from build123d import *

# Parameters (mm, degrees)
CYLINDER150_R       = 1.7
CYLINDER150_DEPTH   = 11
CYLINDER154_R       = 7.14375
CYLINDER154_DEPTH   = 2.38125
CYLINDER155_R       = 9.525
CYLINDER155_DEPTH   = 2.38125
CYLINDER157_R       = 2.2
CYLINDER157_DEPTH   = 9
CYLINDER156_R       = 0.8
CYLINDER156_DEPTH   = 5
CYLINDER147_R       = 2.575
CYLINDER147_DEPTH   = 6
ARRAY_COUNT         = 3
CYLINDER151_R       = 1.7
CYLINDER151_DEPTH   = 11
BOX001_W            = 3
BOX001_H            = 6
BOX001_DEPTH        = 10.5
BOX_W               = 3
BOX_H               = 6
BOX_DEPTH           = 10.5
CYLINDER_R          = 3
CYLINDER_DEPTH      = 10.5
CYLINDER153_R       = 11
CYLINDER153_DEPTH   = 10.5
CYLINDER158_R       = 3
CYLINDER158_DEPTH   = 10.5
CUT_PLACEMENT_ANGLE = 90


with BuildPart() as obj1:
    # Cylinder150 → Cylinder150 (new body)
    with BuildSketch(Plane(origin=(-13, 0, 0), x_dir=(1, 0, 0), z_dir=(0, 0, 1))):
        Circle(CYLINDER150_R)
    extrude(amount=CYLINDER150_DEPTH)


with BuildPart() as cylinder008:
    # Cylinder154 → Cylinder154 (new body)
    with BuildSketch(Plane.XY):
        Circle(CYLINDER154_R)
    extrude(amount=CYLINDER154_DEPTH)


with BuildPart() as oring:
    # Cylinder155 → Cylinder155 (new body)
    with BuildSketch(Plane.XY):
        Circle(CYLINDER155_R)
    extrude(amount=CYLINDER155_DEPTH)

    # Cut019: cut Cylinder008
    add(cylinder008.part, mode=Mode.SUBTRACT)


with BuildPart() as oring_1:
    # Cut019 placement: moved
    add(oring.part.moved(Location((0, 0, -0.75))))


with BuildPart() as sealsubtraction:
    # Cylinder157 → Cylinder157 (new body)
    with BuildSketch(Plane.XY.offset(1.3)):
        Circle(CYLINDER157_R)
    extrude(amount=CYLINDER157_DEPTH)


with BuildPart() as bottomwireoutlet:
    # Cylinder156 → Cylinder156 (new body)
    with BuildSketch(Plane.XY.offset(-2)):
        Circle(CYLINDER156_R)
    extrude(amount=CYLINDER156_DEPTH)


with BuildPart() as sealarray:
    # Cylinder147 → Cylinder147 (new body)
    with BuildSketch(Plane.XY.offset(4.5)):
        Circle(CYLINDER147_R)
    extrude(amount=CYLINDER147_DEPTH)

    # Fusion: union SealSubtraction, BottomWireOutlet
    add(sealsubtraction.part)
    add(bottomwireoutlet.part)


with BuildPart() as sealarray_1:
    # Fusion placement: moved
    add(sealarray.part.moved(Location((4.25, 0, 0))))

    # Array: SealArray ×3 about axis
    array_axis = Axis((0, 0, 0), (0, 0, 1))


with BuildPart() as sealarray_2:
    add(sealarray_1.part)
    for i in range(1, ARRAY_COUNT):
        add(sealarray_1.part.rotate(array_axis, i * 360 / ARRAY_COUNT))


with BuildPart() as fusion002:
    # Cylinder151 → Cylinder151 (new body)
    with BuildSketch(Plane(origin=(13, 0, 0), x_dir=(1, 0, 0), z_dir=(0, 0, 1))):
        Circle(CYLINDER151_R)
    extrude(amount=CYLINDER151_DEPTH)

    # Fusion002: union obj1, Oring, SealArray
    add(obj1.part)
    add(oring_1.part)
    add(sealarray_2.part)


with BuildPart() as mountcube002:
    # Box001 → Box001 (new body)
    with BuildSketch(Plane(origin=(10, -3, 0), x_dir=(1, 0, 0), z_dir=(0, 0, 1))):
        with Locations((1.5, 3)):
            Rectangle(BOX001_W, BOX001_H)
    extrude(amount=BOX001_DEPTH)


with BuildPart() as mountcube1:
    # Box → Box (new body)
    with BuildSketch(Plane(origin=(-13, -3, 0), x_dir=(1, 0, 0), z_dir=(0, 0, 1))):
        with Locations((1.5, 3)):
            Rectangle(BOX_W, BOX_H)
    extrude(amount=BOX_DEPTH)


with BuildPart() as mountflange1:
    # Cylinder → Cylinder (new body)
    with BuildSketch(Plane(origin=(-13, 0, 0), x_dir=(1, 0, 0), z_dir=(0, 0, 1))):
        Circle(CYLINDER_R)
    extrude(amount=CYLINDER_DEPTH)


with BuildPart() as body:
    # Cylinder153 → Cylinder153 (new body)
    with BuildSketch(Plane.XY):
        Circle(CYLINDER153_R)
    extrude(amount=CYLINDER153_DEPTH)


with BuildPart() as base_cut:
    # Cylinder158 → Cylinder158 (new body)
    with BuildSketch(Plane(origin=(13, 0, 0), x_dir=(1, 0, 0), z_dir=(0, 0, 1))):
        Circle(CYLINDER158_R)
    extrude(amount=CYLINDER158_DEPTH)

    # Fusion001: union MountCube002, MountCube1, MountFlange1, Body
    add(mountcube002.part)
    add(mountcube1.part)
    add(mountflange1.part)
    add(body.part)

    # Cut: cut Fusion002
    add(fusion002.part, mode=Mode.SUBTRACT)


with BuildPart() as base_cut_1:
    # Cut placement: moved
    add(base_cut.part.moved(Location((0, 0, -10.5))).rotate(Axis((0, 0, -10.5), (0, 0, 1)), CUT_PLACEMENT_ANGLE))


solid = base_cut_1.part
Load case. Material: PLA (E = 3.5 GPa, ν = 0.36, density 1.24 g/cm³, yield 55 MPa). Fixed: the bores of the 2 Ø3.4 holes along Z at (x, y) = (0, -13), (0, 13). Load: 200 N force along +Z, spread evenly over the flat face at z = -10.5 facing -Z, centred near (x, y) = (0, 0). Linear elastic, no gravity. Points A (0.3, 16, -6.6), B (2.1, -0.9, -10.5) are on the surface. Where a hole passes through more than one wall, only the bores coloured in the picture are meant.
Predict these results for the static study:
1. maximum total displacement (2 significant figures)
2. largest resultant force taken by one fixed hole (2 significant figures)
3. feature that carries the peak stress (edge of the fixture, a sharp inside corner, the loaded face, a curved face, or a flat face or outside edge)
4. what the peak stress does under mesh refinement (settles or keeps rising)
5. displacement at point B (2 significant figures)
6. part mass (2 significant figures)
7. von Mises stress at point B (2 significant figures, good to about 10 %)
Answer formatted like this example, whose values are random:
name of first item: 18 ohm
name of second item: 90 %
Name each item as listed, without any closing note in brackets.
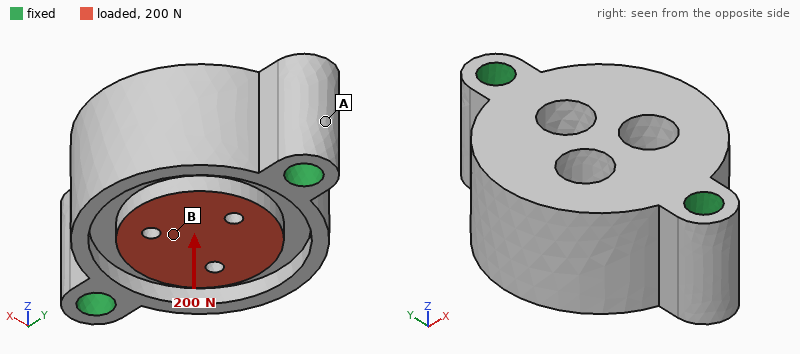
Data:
maximum total displacement: 16 µm
largest resultant force taken by one fixed hole: 100 N
feature that carries the peak stress: edge of the fixture
what the peak stress does under mesh refinement: keeps rising
displacement at point B: 15 µm
part mass: 4.5 g
von Mises stress at point B: 3.1 MPa
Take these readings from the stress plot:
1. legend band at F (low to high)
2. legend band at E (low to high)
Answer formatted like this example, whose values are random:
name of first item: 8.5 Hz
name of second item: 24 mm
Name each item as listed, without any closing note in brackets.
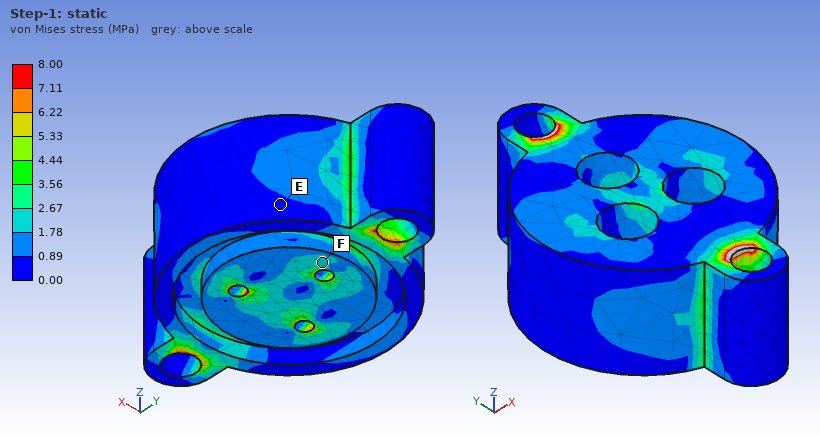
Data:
legend band at F: 1.78 to 2.67 MPa
legend band at E: 0.00 to 0.89 MPa
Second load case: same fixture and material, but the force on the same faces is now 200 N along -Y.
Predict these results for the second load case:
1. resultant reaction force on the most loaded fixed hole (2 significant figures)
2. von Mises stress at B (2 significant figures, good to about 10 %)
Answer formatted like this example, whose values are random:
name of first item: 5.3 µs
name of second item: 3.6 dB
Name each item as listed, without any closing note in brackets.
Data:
resultant reaction force on the most loaded fixed hole: 120 N
von Mises stress at B: 2.8 MPa
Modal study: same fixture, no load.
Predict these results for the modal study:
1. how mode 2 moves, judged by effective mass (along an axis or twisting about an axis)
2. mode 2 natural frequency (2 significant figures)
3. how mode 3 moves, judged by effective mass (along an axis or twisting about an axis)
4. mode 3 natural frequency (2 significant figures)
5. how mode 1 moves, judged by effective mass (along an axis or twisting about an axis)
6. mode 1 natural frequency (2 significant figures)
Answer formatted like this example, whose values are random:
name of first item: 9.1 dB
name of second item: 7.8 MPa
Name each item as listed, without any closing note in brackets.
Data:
how mode 2 moves, judged by effective mass: along Z
mode 2 natural frequency: 11 kHz
how mode 3 moves, judged by effective mass: along X
mode 3 natural frequency: 14 kHz
how mode 1 moves, judged by effective mass: twisting about Y
mode 1 natural frequency: 8700 Hz
